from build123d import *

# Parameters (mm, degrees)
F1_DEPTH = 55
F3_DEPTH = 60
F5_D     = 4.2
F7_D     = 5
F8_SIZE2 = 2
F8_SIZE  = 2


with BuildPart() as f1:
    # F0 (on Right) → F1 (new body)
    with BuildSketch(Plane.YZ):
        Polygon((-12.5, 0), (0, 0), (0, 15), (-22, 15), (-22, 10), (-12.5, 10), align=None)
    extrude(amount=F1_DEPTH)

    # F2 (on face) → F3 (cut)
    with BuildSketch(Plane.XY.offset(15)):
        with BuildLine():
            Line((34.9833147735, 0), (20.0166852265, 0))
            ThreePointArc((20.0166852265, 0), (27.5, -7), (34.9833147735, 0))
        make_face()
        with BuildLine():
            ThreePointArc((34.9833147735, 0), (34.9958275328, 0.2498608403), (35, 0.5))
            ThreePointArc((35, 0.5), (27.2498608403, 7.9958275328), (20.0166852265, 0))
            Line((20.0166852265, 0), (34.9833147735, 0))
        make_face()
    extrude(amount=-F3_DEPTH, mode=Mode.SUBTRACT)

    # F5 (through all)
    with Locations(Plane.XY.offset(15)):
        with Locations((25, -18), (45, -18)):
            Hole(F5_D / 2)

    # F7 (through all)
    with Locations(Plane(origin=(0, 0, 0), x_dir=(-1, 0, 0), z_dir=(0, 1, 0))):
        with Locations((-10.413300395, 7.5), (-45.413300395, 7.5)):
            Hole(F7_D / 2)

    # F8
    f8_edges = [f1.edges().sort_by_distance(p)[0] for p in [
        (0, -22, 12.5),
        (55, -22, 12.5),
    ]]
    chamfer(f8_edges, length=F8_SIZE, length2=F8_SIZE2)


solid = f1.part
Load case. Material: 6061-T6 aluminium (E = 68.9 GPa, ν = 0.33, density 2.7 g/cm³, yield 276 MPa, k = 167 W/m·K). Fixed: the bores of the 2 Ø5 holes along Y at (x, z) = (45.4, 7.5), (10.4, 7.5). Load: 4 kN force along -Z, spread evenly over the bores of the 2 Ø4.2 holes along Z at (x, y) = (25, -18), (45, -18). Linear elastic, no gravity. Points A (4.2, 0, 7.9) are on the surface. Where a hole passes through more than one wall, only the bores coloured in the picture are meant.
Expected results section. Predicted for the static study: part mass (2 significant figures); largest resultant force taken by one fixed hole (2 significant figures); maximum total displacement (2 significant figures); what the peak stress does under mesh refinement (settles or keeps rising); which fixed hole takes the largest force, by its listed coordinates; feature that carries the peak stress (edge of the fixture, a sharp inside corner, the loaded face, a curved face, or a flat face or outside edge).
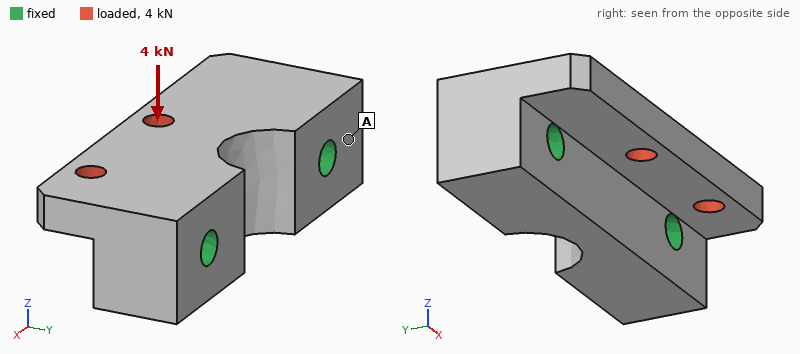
30 g
2.8 kN
73 µm
keeps rising
(45.4, 7.5)
edge of the fixture
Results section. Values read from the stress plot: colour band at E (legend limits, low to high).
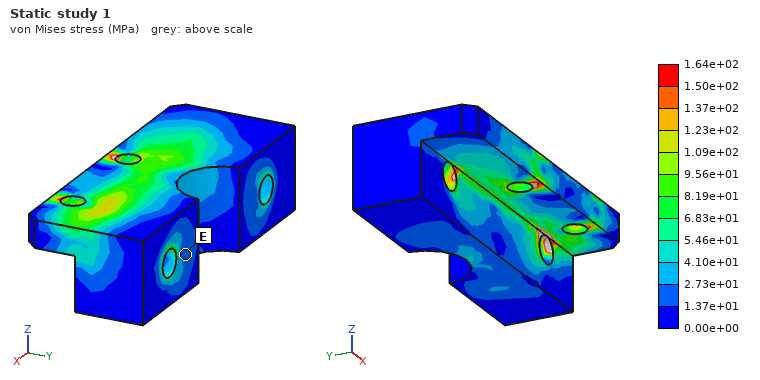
1.37e+01 to 2.73e+01 MPa
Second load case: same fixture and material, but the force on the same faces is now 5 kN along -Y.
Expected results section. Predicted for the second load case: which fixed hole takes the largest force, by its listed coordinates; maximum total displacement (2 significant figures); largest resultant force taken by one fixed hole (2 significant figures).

(45.4, 7.5)
22 µm
3.5 kN
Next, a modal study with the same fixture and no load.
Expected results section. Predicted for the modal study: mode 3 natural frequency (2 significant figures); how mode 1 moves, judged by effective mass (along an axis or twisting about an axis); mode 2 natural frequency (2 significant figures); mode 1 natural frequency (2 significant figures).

29 kHz
along Z
27 kHz
21 kHz
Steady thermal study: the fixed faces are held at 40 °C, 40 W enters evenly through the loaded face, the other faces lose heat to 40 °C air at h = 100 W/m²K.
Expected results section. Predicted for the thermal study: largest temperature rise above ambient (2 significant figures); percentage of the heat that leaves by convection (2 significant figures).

18 K
4.0 %
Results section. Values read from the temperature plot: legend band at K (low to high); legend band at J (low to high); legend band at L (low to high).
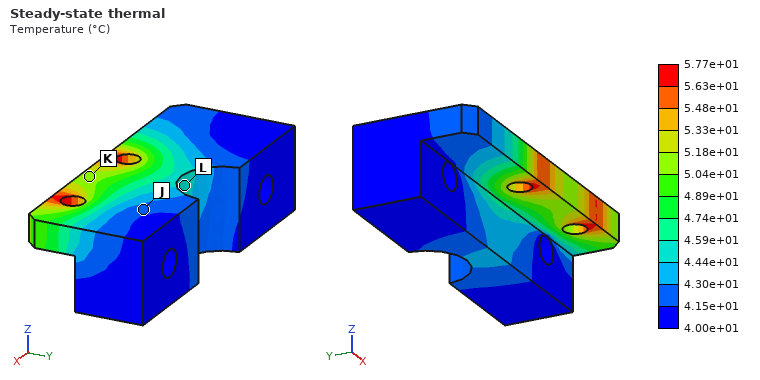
5.04e+01 to 5.18e+01 °C
4.15e+01 to 4.30e+01 °C
4.44e+01 to 4.59e+01 °C
